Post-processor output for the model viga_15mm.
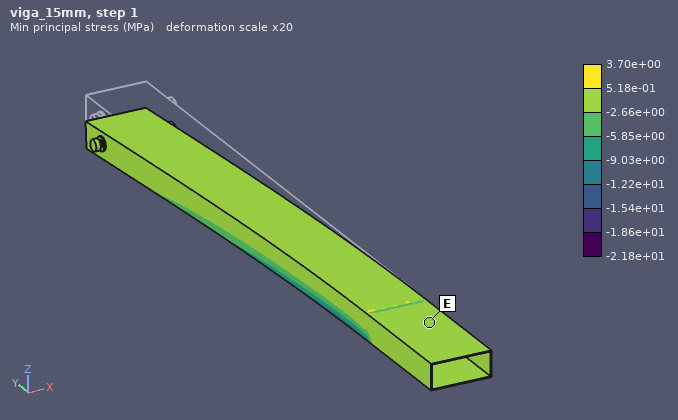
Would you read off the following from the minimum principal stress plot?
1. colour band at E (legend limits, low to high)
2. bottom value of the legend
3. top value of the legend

-2.66e+00 to 5.18e-01 MPa
-2.18e+01 MPa
3.70e+00 MPa
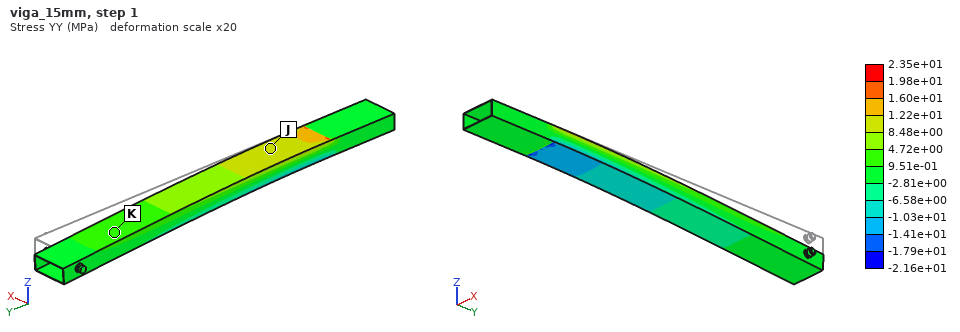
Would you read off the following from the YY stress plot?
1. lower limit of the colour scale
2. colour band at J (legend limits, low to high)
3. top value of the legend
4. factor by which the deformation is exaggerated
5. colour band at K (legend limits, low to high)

-2.16e+01 MPa
8.48e+00 to 1.22e+01 MPa
2.35e+01 MPa
20
9.51e-01 to 4.72e+00 MPa
